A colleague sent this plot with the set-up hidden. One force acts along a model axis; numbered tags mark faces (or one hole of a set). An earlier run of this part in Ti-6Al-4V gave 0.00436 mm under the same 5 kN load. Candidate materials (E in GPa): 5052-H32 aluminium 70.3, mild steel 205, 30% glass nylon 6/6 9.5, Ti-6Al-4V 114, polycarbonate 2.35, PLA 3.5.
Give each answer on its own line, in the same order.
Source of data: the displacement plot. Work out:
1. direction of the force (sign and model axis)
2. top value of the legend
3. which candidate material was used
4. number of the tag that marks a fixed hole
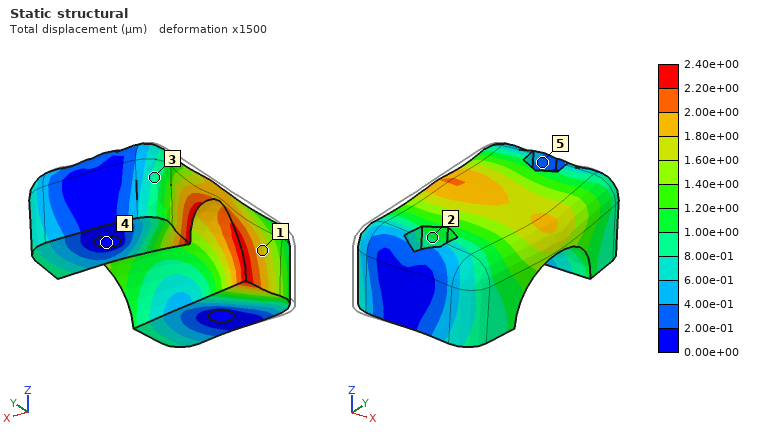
+X
2.40e+00 µm
mild steel
4
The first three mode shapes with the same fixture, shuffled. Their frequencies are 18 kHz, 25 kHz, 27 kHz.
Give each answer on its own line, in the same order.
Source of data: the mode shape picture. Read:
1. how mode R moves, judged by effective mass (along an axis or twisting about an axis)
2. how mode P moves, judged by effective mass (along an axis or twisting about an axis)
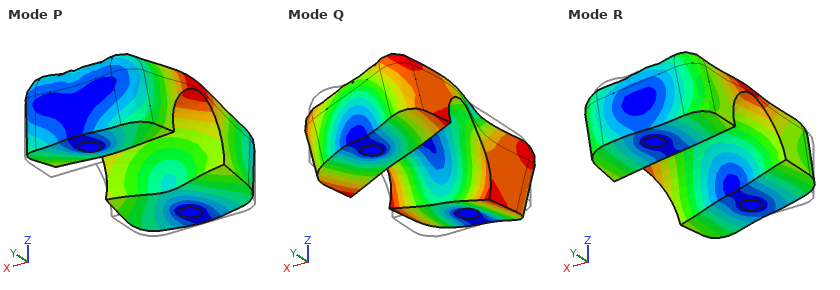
along X
along Z
